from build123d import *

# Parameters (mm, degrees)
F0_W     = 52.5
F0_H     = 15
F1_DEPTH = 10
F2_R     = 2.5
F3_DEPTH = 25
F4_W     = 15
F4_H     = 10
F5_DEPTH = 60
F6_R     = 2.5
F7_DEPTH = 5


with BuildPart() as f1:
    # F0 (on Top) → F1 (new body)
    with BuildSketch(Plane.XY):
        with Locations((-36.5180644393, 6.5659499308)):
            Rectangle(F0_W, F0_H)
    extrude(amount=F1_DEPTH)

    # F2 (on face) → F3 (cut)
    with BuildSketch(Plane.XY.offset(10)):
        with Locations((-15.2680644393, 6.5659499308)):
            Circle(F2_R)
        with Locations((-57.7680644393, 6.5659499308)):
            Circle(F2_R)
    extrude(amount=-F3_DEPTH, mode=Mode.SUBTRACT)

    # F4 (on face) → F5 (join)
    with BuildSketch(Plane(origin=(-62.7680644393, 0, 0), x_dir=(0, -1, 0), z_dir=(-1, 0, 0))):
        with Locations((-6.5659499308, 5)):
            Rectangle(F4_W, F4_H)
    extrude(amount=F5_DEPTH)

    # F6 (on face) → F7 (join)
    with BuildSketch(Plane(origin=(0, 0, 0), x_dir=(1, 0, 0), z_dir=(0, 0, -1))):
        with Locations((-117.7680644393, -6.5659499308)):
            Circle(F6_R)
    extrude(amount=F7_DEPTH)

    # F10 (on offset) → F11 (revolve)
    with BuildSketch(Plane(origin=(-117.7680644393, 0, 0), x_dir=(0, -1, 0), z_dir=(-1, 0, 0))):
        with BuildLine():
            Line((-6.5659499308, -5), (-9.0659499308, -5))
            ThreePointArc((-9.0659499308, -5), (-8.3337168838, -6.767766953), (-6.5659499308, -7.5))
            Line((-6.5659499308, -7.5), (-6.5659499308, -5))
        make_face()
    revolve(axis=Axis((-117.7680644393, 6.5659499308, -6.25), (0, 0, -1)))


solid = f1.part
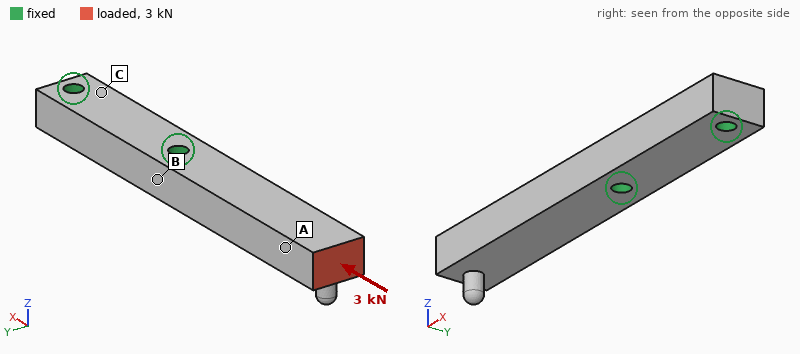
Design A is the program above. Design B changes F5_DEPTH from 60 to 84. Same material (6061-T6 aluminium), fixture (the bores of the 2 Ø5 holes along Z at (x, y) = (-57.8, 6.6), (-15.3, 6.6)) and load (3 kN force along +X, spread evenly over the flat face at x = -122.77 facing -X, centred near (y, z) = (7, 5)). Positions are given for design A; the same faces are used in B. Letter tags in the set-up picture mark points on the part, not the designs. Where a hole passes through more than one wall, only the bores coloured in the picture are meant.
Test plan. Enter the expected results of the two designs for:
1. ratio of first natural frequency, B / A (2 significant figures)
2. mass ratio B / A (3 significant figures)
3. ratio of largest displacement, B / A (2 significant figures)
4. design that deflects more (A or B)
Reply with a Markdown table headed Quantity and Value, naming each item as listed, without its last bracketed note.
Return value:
| Quantity | Value |
|---|---|
| ratio of first natural frequency, B / A | 0.54 |
| mass ratio B / A | 1.22 |
| ratio of largest displacement, B / A | 1.4 |
| design that deflects more | B |
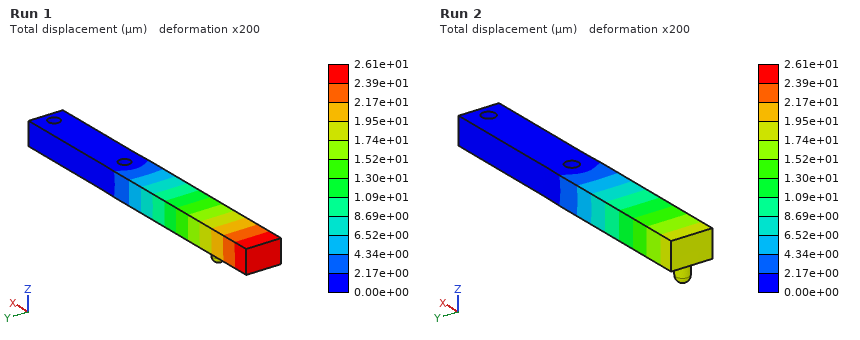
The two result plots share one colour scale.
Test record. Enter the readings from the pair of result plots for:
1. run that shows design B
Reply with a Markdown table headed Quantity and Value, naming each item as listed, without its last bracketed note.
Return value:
| Quantity | Value |
|---|---|
| run that shows design B | Run 1 |
